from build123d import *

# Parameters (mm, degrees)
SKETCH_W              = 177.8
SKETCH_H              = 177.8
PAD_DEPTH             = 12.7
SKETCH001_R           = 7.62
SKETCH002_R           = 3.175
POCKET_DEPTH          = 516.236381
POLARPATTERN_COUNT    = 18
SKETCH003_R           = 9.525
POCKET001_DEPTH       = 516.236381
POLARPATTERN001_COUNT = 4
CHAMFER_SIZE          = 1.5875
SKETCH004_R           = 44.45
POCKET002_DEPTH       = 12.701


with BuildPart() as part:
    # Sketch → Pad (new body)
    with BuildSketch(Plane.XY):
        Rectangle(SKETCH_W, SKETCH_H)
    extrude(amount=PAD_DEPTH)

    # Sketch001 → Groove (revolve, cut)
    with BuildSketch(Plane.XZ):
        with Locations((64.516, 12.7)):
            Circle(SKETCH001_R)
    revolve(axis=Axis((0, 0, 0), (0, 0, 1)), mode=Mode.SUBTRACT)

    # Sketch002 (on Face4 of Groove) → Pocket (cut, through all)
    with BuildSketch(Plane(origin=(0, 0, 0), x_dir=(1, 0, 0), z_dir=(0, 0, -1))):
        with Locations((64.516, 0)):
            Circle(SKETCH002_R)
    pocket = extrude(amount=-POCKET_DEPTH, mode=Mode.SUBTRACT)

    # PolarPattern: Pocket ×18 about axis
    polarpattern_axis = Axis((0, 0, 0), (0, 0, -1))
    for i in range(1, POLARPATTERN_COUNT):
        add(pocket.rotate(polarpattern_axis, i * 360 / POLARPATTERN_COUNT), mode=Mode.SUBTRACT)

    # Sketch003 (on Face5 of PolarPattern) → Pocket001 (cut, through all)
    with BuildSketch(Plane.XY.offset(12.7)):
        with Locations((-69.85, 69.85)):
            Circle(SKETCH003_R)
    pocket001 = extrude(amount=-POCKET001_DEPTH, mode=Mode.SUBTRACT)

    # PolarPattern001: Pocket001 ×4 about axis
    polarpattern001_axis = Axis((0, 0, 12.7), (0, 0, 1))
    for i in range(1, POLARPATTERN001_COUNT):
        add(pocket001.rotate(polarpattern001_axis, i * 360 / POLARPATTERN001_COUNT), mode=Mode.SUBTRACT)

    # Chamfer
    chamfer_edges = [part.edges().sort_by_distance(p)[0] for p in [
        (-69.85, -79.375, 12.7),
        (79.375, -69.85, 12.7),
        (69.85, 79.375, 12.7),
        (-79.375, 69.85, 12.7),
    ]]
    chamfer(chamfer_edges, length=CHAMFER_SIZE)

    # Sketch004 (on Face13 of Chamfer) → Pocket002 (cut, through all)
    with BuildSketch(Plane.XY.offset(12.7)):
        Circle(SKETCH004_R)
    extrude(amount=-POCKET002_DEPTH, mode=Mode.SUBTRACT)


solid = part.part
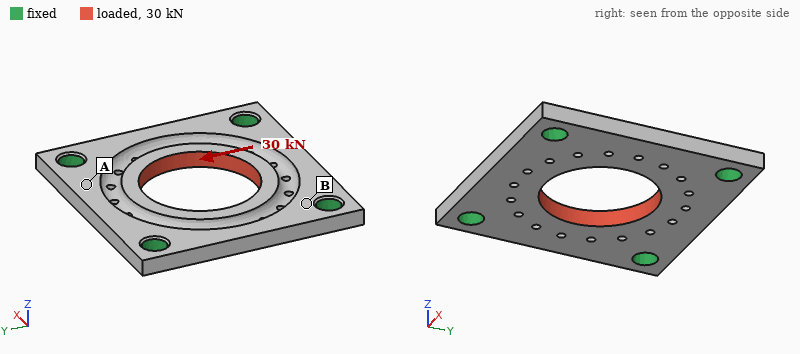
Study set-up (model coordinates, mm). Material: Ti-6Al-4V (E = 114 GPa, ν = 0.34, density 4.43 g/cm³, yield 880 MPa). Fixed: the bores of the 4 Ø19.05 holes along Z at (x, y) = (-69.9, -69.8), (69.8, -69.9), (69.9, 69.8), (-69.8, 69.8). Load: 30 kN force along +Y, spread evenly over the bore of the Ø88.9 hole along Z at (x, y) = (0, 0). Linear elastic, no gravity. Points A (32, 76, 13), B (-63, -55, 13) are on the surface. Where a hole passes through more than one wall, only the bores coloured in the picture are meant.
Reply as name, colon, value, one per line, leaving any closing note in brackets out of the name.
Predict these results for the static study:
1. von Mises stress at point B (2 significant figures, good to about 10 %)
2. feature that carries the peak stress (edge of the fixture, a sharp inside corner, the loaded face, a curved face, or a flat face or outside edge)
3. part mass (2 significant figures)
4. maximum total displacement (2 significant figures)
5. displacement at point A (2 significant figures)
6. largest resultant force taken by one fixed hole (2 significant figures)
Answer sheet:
von Mises stress at point B: 16 MPa
feature that carries the peak stress: a curved face
part mass: 1.2 kg
maximum total displacement: 26 µm
displacement at point A: 8.4 µm
largest resultant force taken by one fixed hole: 7.7 kN
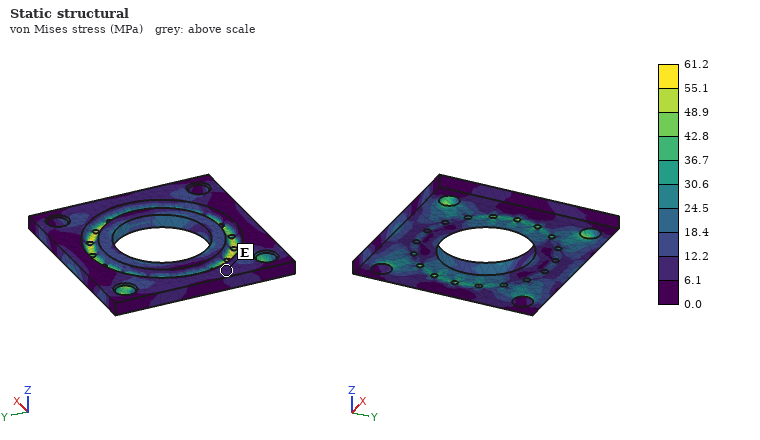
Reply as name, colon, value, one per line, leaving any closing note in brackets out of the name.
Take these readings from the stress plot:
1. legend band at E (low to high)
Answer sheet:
legend band at E: 6.1 to 12.2 MPa
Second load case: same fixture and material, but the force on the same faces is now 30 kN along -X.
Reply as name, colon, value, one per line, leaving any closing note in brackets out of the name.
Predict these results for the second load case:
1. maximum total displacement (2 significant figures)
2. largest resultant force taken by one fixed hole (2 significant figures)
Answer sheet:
maximum total displacement: 26 µm
largest resultant force taken by one fixed hole: 7.7 kN
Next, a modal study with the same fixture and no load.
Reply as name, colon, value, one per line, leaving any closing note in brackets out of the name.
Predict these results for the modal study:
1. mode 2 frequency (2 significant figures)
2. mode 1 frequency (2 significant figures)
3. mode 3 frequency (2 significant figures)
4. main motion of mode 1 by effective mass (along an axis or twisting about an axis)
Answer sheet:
mode 2 frequency: 3900 Hz
mode 1 frequency: 3300 Hz
mode 3 frequency: 3900 Hz
main motion of mode 1 by effective mass: along Z
